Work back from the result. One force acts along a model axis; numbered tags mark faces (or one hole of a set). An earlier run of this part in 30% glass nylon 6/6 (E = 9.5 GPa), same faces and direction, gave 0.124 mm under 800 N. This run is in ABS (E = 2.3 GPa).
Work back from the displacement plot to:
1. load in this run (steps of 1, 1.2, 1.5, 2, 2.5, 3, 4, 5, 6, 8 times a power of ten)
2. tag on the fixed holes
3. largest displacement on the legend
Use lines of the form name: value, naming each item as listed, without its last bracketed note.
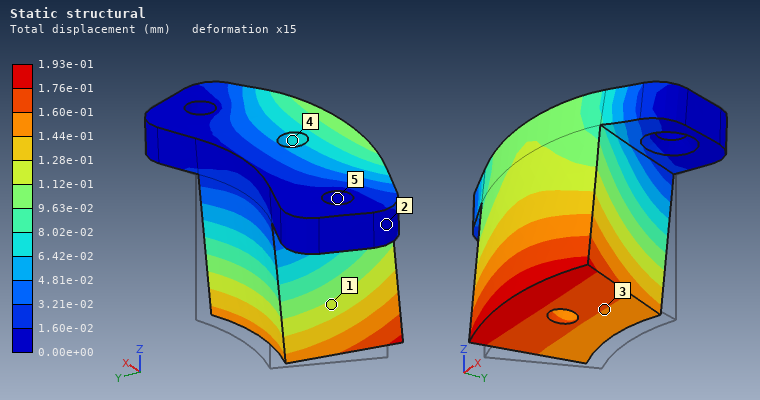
load in this run: 300 N
tag on the fixed holes: 5
largest displacement on the legend: 1.93e-01 mm
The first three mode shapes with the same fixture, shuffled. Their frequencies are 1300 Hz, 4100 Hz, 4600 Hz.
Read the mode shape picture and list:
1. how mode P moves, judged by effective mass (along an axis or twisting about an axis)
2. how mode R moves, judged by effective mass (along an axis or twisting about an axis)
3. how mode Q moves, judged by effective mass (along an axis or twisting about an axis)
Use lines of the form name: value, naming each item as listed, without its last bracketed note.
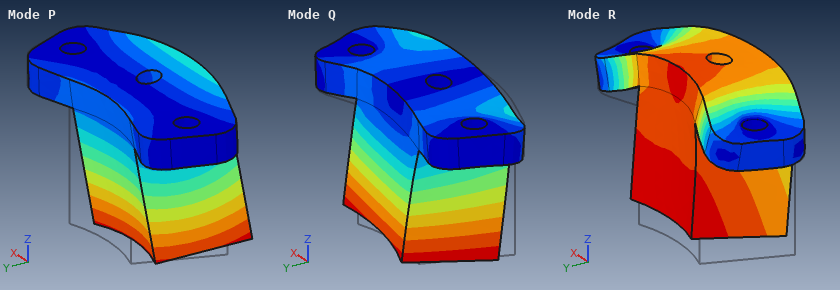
how mode P moves, judged by effective mass: along Y
how mode R moves, judged by effective mass: along Z
how mode Q moves, judged by effective mass: along X
